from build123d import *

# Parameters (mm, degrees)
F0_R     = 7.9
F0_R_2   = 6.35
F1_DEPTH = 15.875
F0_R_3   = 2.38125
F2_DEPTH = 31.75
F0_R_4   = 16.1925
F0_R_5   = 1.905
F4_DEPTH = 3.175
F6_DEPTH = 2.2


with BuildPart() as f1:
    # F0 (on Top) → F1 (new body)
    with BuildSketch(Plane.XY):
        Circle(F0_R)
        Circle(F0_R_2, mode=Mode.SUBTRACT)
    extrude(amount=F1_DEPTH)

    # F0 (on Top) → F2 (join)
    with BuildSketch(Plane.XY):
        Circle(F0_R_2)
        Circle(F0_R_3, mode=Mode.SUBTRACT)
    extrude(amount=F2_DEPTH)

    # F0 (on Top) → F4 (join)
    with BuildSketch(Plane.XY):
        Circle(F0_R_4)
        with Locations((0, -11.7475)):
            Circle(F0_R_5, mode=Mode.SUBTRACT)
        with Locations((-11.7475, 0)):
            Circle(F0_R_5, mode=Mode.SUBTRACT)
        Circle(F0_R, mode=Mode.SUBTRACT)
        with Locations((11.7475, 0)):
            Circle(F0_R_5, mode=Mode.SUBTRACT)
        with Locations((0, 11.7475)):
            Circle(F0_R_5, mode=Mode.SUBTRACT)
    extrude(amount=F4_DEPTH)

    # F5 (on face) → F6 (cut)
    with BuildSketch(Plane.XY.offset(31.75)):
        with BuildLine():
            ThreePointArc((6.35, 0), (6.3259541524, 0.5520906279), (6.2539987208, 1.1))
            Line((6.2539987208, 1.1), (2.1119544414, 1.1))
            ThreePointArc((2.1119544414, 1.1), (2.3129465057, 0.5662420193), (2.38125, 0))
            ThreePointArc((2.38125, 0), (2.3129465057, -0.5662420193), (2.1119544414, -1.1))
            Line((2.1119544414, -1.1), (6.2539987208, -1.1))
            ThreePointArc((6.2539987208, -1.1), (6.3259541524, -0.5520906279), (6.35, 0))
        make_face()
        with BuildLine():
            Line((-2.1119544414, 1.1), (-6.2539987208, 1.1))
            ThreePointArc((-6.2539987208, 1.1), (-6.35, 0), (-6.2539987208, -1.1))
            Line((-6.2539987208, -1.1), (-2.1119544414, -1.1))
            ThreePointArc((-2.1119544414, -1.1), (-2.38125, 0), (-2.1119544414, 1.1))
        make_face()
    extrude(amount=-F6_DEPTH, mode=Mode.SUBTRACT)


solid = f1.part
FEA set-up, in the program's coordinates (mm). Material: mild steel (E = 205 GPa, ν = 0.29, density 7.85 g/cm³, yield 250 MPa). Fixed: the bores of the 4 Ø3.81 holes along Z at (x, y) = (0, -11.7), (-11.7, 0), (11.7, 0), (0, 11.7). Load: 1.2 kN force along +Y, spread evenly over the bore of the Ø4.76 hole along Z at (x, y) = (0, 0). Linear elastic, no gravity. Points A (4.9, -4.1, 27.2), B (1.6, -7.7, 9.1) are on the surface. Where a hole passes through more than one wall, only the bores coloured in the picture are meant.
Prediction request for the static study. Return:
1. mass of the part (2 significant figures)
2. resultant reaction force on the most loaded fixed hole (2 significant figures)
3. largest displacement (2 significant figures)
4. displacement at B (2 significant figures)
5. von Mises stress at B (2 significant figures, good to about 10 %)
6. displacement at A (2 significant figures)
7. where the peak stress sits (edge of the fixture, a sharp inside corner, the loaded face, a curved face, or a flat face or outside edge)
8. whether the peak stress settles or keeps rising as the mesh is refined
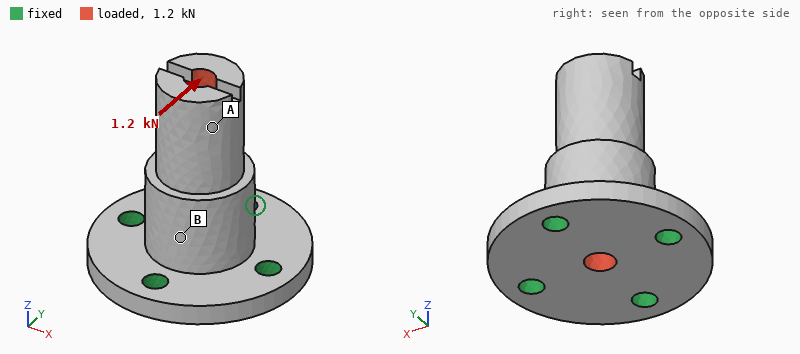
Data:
50 g
930 N
16 µm
4.5 µm
24 MPa
13 µm
edge of the fixture
keeps rising
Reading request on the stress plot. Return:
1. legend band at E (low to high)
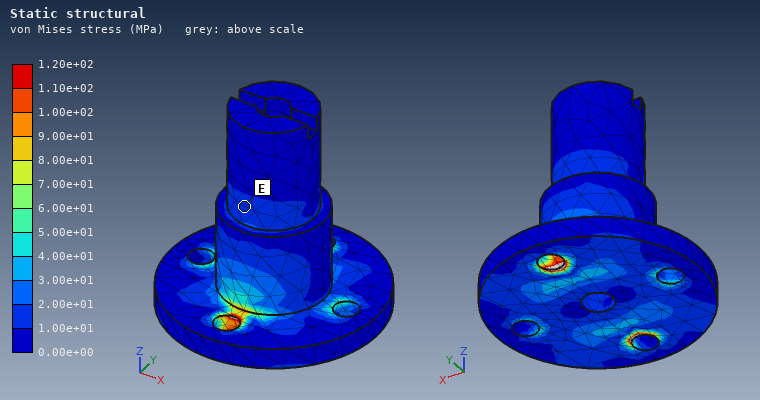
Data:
1.00e+01 to 2.00e+01 MPa
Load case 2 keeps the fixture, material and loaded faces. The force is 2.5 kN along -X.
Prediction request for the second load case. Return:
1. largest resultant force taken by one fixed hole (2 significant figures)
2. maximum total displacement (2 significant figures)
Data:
1.9 kN
34 µm
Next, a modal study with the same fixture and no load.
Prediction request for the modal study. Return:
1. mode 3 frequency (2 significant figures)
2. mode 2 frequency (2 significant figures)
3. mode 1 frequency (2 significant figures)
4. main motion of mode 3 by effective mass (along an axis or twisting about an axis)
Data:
26 kHz
9900 Hz
9800 Hz
along Z
